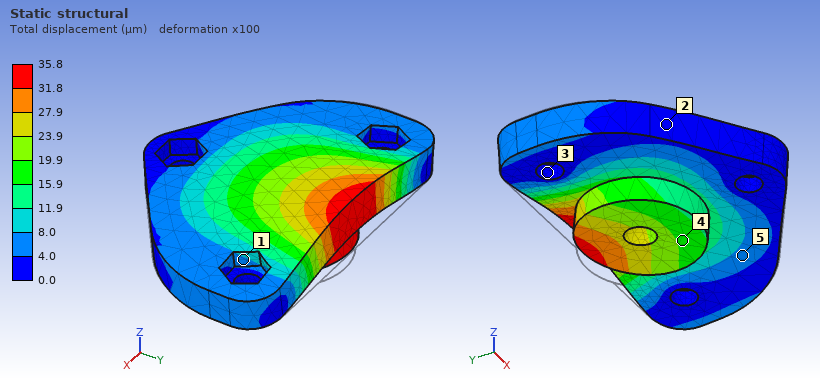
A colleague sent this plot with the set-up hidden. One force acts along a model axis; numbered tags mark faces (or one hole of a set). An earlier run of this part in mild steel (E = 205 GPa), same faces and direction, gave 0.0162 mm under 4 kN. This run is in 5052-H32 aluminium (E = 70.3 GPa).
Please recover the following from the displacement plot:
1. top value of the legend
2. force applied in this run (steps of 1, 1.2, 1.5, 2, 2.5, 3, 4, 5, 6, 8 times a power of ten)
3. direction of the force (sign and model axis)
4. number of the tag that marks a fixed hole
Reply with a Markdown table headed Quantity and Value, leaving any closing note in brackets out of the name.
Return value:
| Quantity | Value |
|---|---|
| top value of the legend | 35.8 µm |
| force applied in this run | 3 kN |
| direction of the force | +Z |
| number of the tag that marks a fixed hole | 3 |
